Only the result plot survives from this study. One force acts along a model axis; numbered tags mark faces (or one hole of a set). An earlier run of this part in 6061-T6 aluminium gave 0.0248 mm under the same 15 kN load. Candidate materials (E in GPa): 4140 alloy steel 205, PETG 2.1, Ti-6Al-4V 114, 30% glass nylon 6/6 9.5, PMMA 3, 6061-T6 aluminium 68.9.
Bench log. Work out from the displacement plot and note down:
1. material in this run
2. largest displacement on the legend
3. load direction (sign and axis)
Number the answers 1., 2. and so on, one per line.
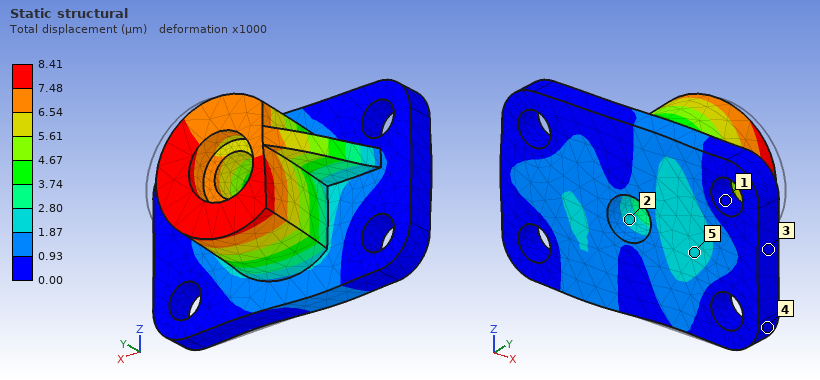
1. 4140 alloy steel
2. 8.41 µm
3. -X
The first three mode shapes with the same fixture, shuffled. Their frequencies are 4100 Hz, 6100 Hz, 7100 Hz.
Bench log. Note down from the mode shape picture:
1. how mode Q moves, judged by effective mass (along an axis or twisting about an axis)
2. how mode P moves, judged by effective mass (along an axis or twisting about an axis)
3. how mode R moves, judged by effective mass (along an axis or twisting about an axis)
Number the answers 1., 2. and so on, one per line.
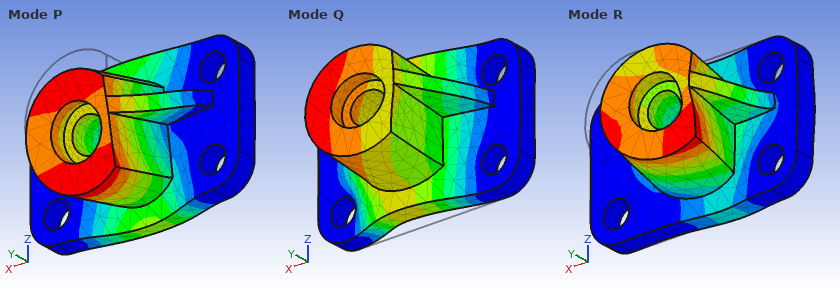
1. along Y
2. along Z
3. along X
